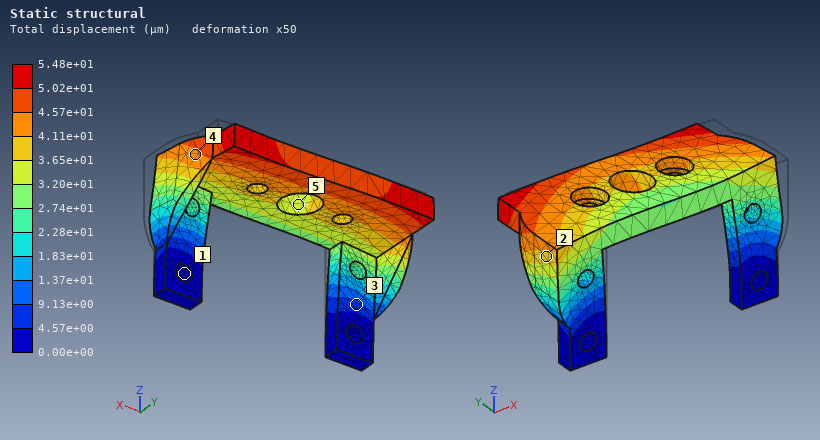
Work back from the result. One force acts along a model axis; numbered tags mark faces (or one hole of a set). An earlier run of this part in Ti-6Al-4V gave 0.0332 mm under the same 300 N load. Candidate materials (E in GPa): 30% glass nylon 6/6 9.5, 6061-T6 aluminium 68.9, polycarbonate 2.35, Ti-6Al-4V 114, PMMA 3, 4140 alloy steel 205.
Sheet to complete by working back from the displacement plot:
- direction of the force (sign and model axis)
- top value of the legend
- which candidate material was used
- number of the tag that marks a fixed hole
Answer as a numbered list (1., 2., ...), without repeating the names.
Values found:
1. -X
2. 5.48e+01 µm
3. 6061-T6 aluminium
4. 1
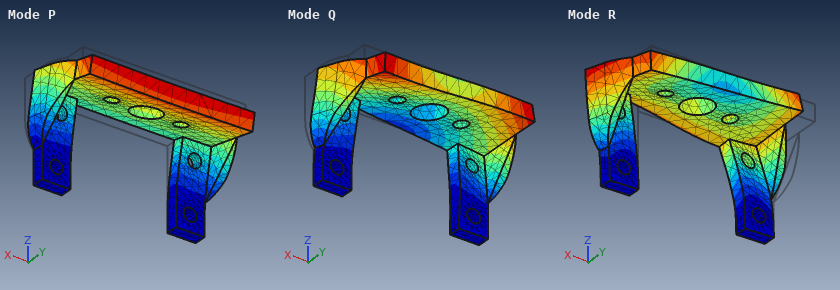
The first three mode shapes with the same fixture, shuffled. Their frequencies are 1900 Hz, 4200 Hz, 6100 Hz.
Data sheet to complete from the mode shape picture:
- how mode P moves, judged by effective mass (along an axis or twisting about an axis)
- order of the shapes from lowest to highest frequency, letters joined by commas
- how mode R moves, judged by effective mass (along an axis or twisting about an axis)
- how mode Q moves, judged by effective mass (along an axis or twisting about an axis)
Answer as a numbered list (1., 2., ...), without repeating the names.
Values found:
1. along Y
2. P, Q, R
3. along X
4. along X
